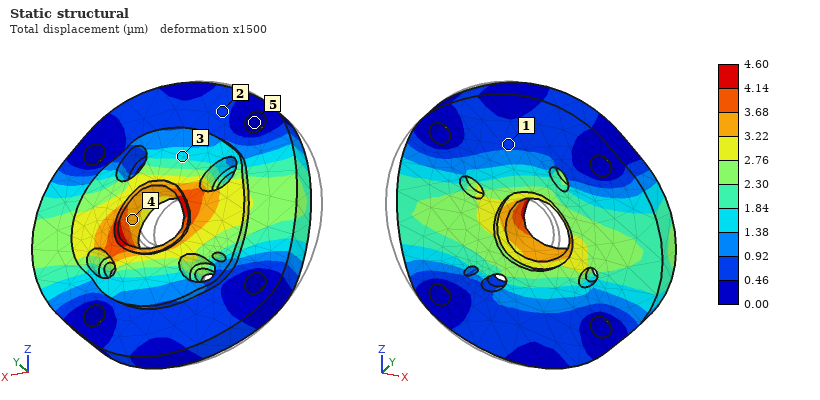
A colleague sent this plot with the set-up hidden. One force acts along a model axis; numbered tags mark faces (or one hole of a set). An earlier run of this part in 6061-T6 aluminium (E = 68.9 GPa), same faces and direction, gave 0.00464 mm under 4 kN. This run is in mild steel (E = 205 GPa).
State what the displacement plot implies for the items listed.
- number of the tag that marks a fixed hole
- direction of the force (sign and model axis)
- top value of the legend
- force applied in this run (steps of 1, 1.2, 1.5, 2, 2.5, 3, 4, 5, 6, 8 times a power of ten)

5
+X
4.60 µm
12 kN
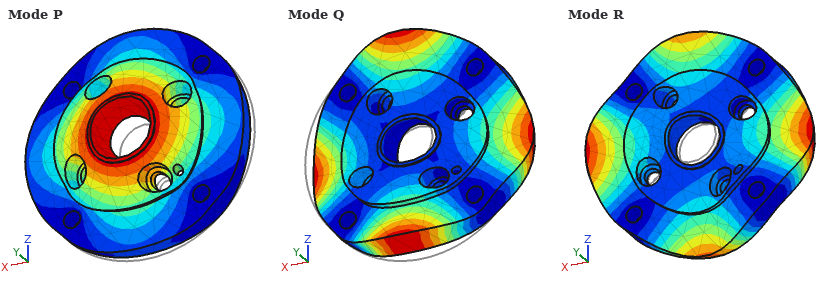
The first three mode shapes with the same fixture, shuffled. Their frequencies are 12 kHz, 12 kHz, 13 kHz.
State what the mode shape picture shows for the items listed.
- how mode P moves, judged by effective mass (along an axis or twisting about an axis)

along Y
